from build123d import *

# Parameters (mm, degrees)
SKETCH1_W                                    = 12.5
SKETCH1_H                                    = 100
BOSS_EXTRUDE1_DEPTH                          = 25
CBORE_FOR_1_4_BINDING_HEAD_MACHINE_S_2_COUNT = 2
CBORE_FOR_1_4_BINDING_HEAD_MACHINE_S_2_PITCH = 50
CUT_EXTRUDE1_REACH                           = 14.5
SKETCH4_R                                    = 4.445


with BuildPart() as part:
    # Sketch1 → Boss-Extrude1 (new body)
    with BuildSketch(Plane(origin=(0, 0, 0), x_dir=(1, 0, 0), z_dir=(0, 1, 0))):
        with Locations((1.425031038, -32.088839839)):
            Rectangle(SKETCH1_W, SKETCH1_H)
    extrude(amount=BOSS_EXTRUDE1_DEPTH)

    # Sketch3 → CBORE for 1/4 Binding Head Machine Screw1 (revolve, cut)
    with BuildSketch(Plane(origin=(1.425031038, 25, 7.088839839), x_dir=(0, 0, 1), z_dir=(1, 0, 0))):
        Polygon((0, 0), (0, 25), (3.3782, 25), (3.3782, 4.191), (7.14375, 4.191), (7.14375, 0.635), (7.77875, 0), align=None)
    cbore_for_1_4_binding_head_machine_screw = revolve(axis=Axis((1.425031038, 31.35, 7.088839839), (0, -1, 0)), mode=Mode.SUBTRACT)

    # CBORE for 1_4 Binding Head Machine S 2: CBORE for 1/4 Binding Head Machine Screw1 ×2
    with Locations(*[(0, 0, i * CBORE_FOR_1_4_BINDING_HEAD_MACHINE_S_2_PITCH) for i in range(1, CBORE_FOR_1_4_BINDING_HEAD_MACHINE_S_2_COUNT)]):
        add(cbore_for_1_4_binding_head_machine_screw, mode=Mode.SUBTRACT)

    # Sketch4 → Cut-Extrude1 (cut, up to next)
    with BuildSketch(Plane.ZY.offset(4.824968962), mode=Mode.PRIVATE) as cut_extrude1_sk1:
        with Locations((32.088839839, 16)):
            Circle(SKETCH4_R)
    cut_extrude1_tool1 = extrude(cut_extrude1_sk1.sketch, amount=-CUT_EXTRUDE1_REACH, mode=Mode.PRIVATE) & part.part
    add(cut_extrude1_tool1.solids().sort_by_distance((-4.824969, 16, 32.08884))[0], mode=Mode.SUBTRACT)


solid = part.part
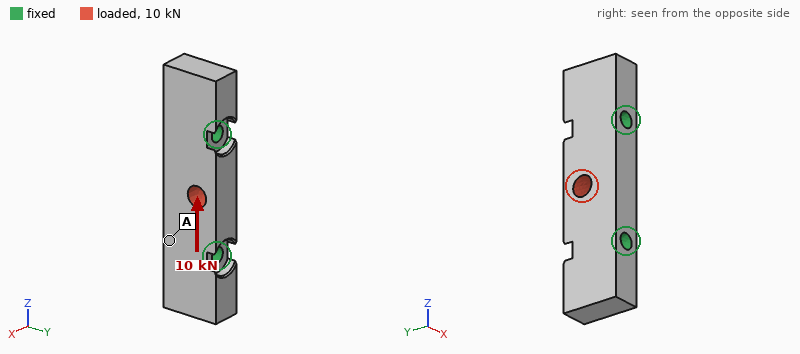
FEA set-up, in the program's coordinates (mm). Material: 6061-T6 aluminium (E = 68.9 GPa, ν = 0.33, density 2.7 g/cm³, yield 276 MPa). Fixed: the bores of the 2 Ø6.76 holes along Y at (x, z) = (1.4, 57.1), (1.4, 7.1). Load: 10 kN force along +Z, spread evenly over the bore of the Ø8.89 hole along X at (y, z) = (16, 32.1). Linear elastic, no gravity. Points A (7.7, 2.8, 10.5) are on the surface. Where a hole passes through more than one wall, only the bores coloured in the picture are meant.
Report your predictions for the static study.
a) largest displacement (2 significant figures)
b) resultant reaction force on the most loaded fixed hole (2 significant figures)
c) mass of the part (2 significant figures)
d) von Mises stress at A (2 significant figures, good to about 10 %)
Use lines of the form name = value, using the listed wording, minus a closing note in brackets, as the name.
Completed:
largest displacement = 9.2 µm
resultant reaction force on the most loaded fixed hole = 5.1 kN
mass of the part = 75 g
von Mises stress at A = 7.6 MPa
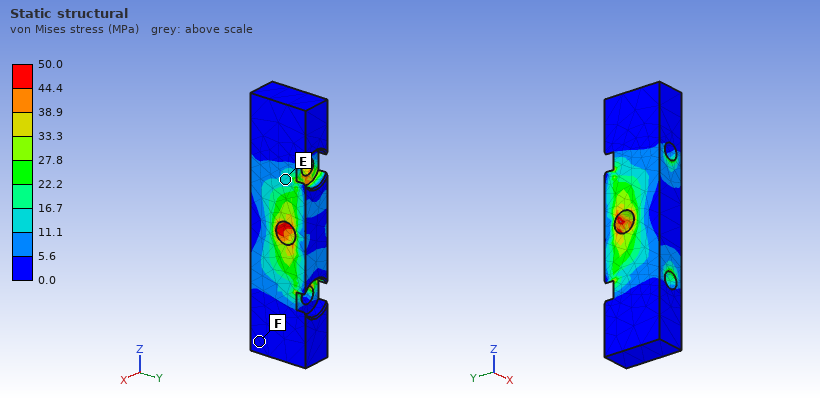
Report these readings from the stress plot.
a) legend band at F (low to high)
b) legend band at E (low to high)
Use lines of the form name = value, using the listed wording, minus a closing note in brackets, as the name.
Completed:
legend band at F = 0.0 to 5.6 MPa
legend band at E = 11.1 to 16.7 MPa
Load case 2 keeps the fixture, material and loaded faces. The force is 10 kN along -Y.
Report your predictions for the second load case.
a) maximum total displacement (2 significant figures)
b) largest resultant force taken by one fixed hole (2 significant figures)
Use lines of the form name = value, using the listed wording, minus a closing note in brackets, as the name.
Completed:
maximum total displacement = 26 µm
largest resultant force taken by one fixed hole = 5.1 kN
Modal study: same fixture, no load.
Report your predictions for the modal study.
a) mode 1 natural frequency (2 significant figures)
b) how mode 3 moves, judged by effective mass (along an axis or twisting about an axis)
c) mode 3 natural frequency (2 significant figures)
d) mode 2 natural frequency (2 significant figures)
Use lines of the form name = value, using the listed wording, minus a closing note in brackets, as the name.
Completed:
mode 1 natural frequency = 13 kHz
how mode 3 moves, judged by effective mass = along X
mode 3 natural frequency = 19 kHz
mode 2 natural frequency = 13 kHz
